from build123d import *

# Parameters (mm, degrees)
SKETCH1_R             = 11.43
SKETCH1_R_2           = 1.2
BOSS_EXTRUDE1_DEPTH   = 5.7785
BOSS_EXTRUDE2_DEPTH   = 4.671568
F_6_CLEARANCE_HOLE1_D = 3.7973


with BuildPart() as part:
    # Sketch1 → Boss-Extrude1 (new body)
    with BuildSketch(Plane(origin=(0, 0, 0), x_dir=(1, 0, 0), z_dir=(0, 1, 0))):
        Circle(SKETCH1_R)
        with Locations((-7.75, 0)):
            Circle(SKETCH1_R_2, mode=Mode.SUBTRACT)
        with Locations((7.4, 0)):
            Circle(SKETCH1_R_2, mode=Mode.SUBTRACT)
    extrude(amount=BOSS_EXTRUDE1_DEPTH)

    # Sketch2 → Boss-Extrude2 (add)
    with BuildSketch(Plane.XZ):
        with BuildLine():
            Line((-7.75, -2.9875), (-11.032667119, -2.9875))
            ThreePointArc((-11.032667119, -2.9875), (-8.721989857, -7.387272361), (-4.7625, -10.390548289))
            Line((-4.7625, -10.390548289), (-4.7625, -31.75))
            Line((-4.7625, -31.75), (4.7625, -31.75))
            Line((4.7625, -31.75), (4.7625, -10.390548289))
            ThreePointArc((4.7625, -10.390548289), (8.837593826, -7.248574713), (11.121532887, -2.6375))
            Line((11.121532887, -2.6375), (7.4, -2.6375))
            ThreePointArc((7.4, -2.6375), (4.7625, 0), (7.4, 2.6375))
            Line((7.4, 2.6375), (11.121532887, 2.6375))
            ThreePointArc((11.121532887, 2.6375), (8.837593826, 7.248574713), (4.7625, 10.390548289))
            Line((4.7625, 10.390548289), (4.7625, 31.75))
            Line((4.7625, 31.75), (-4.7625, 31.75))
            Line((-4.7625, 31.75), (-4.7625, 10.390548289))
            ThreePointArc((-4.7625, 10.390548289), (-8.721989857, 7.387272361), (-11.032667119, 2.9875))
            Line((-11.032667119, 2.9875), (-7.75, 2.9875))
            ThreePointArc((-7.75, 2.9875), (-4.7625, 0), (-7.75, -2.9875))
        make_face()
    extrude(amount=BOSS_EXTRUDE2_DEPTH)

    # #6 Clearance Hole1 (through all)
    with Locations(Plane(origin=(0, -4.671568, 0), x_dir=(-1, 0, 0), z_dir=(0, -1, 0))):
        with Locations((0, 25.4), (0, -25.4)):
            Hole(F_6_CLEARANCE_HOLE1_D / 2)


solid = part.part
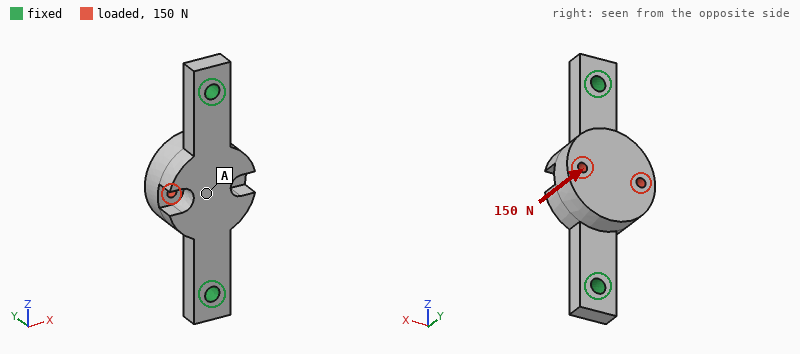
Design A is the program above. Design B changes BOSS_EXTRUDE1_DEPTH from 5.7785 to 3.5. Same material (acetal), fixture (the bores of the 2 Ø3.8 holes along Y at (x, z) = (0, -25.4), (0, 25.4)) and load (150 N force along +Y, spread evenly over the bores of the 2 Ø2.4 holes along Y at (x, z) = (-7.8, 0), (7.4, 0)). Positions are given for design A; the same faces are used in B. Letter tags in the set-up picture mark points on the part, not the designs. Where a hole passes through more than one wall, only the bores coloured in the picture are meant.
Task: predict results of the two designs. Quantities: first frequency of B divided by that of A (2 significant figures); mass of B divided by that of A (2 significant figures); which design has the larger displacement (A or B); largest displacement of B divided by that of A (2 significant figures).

1.3
0.84
B
1.2
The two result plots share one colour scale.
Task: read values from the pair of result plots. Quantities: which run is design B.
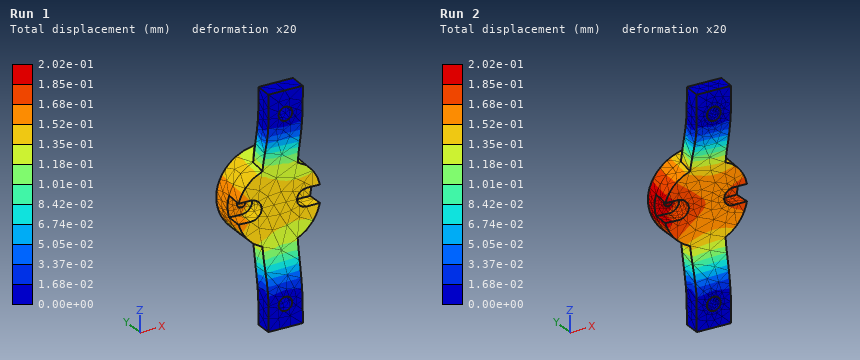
Run 2
